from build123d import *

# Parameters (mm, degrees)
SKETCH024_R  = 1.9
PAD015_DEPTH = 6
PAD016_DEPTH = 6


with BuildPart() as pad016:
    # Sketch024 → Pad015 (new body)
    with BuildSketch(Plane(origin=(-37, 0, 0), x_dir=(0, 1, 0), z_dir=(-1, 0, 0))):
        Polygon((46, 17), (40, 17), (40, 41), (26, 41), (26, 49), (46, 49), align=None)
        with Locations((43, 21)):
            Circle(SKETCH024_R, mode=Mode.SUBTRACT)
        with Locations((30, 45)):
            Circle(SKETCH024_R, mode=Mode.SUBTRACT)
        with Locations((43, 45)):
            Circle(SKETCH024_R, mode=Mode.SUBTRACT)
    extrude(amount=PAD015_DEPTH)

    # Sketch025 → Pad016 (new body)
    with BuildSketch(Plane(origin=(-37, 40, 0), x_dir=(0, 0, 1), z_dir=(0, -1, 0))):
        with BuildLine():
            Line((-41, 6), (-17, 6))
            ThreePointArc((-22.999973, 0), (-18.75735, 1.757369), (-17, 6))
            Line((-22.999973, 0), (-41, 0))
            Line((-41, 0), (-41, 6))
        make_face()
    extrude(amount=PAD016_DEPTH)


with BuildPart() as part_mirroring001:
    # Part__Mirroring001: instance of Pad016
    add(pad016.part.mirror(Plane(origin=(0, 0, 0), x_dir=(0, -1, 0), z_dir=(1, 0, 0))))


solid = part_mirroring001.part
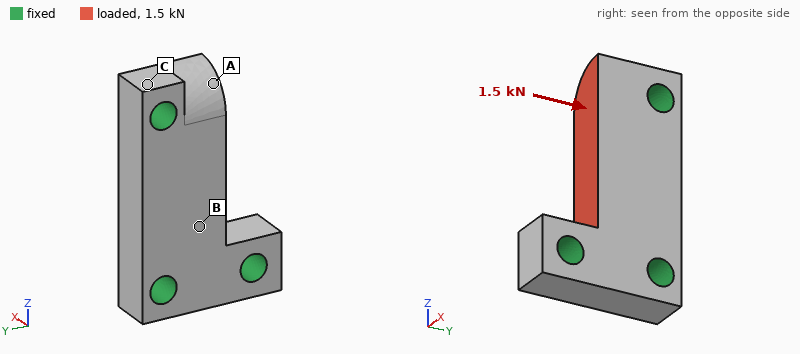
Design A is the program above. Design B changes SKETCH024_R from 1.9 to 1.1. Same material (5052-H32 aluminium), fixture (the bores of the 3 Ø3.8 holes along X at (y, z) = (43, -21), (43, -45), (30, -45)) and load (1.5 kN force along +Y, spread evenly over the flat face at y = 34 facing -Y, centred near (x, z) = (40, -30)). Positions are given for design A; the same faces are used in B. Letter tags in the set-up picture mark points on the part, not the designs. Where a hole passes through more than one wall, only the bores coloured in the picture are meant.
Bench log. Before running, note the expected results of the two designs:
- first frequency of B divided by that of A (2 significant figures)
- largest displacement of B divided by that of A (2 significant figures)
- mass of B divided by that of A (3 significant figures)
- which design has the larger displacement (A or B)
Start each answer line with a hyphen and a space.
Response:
- 0.86
- 1.2
- 1.06
- B
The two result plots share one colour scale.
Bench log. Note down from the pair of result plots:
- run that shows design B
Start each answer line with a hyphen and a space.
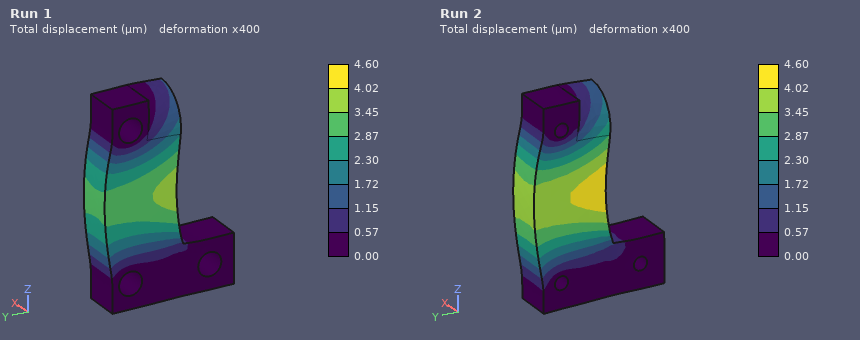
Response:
- Run 2
